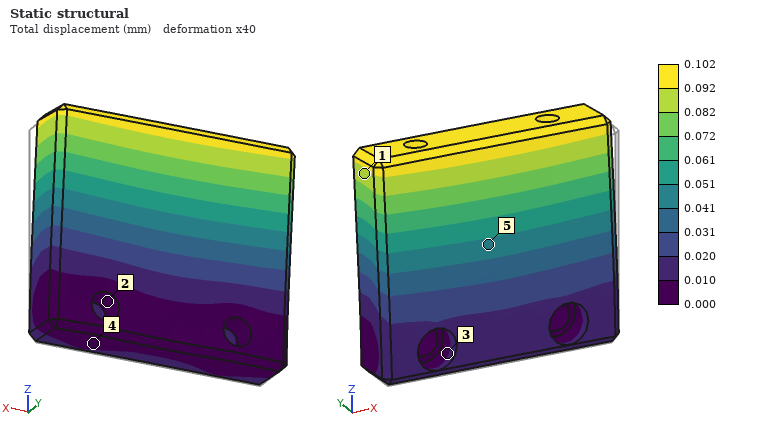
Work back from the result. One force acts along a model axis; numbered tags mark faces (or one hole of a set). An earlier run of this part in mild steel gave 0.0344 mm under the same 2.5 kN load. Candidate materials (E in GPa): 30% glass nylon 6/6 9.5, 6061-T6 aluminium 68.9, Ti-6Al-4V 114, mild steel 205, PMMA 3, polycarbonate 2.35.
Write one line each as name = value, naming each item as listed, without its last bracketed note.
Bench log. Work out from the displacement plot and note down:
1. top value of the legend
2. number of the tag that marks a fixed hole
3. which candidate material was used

top value of the legend = 0.102 mm
number of the tag that marks a fixed hole = 2
which candidate material was used = 6061-T6 aluminium
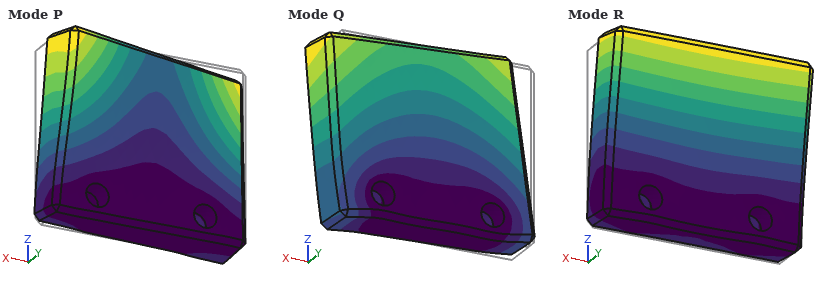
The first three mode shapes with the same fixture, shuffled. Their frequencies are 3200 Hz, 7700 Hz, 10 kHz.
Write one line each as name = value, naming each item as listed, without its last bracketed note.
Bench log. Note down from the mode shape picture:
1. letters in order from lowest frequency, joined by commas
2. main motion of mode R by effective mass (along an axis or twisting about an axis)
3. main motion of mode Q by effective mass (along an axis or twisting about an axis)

letters in order from lowest frequency, joined by commas = R, P, Q
main motion of mode R by effective mass = along Y
main motion of mode Q by effective mass = along X
